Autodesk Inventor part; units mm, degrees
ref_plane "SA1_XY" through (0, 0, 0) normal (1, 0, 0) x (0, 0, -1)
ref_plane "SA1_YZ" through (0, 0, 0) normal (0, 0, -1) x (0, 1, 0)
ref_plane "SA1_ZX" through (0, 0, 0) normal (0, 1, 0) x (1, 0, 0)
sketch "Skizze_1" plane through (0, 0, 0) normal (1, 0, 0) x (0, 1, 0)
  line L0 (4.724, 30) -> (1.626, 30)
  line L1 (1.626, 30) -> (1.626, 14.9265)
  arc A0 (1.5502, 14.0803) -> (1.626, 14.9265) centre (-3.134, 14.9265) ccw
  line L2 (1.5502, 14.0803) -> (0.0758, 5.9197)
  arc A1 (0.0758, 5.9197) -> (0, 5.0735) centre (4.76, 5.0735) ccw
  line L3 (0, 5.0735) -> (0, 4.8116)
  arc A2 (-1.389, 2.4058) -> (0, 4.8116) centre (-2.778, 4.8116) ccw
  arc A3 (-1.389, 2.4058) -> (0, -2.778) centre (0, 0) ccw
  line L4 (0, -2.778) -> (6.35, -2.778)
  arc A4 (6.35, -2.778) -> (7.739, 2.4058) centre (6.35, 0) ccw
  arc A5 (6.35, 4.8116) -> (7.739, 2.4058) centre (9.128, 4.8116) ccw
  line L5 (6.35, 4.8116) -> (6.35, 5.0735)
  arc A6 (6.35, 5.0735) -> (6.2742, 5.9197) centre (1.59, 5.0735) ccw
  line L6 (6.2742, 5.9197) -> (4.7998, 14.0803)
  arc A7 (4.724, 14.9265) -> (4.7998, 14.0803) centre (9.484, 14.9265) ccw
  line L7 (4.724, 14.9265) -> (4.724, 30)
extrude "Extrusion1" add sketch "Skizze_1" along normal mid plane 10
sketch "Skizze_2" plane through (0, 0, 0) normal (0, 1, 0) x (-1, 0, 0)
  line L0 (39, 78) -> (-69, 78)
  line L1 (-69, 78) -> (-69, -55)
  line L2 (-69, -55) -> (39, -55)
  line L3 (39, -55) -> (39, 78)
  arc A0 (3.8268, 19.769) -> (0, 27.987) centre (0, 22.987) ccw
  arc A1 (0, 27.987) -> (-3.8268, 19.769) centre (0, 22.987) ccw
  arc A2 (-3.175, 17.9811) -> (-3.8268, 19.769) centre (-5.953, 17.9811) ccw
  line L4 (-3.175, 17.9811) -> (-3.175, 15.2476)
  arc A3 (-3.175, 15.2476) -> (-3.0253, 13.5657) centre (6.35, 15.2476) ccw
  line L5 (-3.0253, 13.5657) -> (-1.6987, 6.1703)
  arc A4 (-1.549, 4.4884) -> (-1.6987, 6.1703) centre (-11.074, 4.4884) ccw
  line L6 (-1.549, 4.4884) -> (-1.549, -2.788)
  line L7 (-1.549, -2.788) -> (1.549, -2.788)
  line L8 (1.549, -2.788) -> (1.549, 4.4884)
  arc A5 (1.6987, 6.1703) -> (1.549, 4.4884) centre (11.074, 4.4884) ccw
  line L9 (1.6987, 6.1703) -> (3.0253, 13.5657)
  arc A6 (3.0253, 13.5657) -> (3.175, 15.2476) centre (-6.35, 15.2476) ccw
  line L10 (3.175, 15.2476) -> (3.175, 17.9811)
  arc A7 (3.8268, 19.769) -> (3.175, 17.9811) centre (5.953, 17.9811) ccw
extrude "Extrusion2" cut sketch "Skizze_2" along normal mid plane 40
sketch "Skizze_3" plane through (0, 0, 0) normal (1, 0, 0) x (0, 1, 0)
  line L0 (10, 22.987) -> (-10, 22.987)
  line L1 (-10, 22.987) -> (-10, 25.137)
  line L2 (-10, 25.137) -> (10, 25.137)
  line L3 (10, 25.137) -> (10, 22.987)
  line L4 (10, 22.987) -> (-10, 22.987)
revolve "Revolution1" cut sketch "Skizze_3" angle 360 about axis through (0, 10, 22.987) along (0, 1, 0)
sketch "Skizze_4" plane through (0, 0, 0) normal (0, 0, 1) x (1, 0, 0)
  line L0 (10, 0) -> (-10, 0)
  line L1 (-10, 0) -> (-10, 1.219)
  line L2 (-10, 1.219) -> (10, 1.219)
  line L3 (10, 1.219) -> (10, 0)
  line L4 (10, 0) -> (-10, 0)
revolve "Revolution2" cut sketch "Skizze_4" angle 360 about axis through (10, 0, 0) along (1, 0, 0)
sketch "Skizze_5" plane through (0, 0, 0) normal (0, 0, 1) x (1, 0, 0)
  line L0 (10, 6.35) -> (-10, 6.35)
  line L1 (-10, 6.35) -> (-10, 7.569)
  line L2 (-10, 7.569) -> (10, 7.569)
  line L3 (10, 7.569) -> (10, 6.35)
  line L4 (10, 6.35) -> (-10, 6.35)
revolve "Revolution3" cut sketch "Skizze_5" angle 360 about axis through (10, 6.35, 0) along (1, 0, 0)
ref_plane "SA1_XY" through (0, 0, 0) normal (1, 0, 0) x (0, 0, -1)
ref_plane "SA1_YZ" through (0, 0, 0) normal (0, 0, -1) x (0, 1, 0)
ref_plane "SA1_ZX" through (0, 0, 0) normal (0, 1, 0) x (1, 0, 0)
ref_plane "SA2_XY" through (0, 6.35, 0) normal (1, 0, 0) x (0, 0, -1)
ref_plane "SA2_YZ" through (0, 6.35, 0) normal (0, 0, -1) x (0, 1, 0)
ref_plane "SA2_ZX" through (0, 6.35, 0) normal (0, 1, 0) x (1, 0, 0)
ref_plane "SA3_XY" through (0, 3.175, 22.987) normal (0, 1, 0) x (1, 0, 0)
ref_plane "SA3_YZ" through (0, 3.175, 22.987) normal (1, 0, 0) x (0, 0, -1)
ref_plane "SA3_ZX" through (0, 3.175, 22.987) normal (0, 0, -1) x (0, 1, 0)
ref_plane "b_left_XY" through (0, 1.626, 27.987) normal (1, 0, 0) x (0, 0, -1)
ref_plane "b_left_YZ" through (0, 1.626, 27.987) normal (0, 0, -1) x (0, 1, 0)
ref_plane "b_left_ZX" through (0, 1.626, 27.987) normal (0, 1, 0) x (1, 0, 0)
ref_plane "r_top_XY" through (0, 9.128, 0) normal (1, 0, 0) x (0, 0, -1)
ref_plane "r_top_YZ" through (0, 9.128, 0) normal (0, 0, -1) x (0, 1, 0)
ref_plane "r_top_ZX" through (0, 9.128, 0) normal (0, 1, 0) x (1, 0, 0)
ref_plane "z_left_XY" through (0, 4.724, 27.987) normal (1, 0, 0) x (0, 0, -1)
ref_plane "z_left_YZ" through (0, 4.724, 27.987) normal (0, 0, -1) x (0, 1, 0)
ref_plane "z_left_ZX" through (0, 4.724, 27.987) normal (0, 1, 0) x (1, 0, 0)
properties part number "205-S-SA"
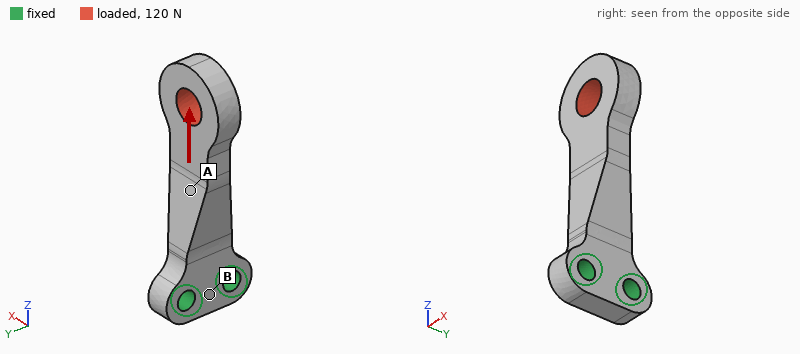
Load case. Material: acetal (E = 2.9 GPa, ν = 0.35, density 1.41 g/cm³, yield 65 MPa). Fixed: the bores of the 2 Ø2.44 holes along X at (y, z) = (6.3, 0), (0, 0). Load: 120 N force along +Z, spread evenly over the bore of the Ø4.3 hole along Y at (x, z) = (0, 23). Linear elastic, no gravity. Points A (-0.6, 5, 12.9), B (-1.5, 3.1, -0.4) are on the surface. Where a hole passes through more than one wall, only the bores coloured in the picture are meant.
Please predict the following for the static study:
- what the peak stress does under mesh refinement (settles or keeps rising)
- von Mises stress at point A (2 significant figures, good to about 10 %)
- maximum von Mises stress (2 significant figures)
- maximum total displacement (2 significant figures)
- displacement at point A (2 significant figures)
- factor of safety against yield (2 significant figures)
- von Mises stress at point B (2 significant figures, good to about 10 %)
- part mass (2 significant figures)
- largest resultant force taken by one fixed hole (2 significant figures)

settles
6.0 MPa
14 MPa
60 µm
23 µm
4.5
1.5 MPa
0.96 g
64 N
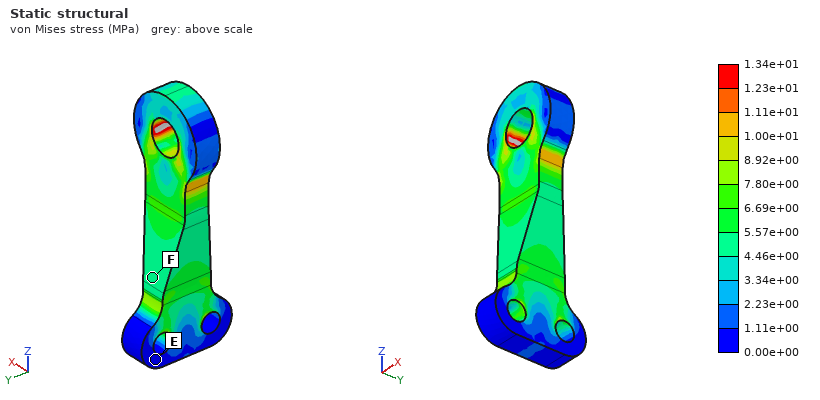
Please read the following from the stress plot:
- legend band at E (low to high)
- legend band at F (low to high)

0.00e+00 to 1.11e+00 MPa
4.46e+00 to 5.57e+00 MPa
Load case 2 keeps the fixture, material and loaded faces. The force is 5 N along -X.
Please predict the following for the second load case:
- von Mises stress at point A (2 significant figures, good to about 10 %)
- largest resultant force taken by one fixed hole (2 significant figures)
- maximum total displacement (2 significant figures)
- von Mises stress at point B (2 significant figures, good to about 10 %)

1.3 MPa
2.5 N
0.37 mm
2.0 MPa
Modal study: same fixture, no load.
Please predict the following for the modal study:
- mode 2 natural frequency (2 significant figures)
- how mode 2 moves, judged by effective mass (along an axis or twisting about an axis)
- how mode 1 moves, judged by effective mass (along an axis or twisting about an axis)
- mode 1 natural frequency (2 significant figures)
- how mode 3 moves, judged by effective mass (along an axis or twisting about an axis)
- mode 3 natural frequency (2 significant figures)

1700 Hz
along Y
along X
1100 Hz
twisting about Z
5200 Hz
